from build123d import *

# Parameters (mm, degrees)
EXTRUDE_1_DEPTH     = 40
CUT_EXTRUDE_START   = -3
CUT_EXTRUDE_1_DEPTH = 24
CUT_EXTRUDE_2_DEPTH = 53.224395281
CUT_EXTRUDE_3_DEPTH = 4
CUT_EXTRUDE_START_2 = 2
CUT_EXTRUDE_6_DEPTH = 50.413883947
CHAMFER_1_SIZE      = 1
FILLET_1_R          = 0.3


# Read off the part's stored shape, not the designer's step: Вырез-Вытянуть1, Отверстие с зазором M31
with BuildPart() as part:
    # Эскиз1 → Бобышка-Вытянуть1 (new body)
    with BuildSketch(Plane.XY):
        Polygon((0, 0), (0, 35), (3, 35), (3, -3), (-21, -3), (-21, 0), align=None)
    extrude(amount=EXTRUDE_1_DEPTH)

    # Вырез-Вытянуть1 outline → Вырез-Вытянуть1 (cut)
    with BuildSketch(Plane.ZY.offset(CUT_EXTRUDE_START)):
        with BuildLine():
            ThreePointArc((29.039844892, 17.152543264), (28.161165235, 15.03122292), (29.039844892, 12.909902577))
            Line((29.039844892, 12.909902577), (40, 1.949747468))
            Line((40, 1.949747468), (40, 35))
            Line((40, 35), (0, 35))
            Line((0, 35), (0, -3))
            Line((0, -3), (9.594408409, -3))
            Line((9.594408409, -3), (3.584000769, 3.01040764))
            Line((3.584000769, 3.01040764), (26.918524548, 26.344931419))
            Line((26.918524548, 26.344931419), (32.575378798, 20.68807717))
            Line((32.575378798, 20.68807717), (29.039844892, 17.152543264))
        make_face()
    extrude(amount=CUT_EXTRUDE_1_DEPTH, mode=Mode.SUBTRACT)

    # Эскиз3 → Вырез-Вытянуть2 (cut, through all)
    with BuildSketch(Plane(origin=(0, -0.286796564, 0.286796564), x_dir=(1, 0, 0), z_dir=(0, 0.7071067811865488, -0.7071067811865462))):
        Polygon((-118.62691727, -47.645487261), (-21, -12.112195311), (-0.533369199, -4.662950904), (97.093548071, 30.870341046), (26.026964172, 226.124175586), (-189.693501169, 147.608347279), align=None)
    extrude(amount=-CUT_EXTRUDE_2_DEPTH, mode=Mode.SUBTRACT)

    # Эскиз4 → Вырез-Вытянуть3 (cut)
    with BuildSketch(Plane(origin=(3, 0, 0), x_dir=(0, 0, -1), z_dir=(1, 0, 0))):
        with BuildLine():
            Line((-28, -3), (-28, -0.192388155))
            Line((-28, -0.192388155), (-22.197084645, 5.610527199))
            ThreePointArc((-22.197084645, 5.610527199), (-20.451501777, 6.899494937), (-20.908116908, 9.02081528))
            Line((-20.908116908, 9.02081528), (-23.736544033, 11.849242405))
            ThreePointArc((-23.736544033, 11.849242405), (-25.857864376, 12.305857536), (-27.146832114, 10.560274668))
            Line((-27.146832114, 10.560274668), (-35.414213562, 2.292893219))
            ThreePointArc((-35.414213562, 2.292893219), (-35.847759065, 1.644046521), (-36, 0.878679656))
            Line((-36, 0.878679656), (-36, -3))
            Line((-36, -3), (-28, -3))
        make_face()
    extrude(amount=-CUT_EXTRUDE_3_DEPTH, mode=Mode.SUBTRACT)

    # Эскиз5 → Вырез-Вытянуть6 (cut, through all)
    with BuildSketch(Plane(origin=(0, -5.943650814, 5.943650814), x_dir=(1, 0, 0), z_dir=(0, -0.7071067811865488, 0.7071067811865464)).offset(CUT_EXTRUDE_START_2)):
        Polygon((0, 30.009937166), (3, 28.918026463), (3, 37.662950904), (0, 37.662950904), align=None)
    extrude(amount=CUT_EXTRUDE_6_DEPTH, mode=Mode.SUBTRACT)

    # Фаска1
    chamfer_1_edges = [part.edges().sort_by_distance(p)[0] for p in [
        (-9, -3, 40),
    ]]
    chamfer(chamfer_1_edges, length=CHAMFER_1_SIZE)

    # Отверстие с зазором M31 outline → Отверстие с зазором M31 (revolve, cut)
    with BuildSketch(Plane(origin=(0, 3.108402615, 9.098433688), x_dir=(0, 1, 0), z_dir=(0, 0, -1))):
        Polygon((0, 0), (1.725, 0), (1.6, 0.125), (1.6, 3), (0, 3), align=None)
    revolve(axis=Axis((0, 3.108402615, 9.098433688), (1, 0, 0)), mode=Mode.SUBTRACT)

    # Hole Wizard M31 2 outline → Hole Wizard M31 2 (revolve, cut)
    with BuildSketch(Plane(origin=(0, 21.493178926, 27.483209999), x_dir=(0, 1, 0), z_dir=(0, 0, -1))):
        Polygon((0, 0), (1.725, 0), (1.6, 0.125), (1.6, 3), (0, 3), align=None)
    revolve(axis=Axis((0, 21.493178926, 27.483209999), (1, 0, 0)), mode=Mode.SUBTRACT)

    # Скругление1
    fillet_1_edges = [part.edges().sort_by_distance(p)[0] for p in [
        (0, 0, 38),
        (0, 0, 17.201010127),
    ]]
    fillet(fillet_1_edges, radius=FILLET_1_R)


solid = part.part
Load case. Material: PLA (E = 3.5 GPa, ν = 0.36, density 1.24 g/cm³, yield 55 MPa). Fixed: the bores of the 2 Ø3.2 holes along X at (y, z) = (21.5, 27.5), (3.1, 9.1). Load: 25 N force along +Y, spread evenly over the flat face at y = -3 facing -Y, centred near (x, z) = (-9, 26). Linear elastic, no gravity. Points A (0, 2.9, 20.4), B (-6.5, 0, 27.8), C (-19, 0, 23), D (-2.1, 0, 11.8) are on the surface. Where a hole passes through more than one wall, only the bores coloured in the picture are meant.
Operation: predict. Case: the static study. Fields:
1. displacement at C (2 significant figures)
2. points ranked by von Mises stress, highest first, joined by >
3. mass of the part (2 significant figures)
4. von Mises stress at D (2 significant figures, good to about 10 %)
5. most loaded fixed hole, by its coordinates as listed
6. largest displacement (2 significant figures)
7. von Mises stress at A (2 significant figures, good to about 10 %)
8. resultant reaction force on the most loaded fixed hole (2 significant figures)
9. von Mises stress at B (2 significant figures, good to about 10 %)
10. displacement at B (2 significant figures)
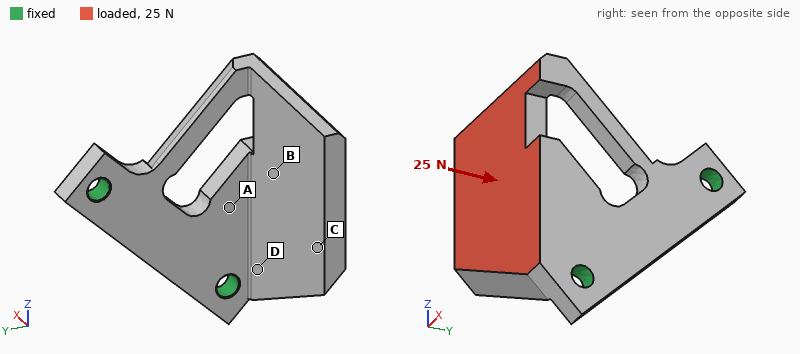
0.44 mm
A > D > B > C
3.7 g
6.3 MPa
(21.5, 27.5)
0.60 mm
8.0 MPa
18 N
2.8 MPa
0.19 mm
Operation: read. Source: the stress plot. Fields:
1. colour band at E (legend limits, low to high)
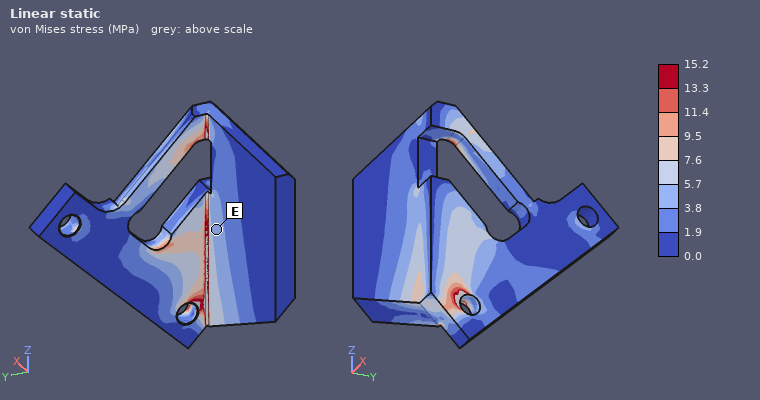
3.8 to 5.7 MPa
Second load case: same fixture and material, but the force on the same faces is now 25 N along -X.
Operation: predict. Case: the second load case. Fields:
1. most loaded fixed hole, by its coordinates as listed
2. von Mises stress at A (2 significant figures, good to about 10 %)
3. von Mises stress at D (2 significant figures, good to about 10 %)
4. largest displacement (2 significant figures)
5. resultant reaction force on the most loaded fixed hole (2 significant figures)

(3.1, 9.1)
3.3 MPa
4.3 MPa
0.55 mm
22 N
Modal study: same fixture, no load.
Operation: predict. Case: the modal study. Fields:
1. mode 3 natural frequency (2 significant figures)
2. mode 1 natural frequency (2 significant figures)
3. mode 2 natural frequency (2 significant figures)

3200 Hz
760 Hz
1100 Hz
